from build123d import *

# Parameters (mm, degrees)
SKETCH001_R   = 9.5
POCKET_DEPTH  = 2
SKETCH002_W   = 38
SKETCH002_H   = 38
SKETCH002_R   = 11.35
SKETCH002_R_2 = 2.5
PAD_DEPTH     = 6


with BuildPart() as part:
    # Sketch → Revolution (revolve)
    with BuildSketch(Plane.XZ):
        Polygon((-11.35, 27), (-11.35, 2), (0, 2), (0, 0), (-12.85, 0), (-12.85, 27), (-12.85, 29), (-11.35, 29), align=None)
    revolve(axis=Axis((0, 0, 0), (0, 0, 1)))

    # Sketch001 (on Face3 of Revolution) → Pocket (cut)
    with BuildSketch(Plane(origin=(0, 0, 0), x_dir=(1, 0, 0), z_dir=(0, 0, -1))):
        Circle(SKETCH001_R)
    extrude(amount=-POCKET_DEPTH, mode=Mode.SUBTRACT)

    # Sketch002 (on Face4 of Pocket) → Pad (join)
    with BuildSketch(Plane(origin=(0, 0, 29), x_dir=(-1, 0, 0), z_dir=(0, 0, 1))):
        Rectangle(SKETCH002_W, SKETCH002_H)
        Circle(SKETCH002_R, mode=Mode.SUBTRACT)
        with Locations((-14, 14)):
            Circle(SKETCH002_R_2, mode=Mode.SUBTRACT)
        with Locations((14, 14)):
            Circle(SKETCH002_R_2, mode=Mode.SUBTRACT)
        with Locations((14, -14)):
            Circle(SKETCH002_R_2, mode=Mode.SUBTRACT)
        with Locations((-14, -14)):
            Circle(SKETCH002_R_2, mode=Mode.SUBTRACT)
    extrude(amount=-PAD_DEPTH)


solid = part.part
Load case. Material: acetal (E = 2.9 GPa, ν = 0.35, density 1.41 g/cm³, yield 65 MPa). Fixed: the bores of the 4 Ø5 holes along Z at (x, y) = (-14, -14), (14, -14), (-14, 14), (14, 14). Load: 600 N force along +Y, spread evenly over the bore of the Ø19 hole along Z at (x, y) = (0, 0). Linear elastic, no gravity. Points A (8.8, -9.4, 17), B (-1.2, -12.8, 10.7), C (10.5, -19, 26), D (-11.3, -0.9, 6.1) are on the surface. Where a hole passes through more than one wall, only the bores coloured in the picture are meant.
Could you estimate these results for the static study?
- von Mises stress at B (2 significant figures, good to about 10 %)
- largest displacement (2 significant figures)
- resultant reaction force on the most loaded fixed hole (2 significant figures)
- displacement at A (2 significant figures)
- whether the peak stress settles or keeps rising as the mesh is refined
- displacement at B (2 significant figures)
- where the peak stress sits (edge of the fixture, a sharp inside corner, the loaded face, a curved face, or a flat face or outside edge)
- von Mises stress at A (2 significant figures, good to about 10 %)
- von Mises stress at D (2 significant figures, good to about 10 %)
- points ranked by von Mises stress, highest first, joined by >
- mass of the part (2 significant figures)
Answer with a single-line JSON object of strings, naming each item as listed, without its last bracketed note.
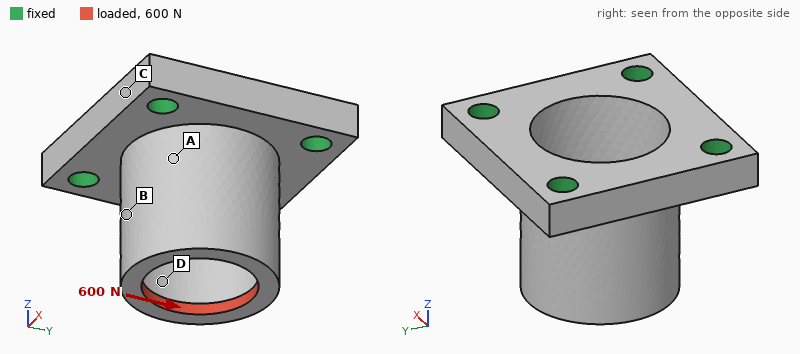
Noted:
{"von Mises stress at B": "8.9 MPa", "largest displacement": "0.58 mm", "resultant reaction force on the most loaded fixed hole": "360 N", "displacement at A": "0.15 mm", "whether the peak stress settles or keeps rising as the mesh is refined": "keeps rising", "displacement at B": "0.31 mm", "where the peak stress sits": "edge of the fixture", "von Mises stress at A": "13 MPa", "von Mises stress at D": "21 MPa", "points ranked by von Mises stress, highest first, joined by >": "D > A > B > C", "mass of the part": "12 g"}
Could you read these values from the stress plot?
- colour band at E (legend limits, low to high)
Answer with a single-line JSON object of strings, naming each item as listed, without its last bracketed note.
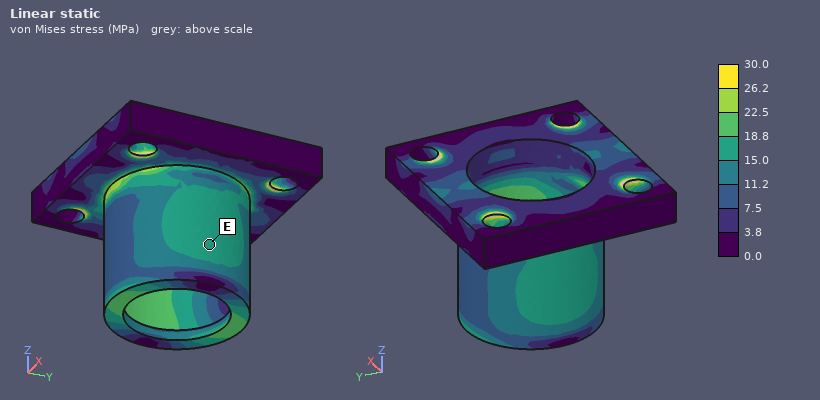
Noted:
{"colour band at E": "15.0 to 18.8 MPa"}
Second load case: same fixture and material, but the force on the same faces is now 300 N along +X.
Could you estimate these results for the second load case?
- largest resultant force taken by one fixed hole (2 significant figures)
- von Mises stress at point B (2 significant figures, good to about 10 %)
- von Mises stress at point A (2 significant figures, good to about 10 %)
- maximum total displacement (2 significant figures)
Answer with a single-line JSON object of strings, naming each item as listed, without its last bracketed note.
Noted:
{"largest resultant force taken by one fixed hole": "180 N", "von Mises stress at point B": "8.9 MPa", "von Mises stress at point A": "6.8 MPa", "maximum total displacement": "0.29 mm"}
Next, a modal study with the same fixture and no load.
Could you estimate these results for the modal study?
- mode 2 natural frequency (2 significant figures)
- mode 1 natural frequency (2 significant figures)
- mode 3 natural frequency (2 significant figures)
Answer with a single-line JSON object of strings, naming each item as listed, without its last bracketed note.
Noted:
{"mode 2 natural frequency": "4000 Hz", "mode 1 natural frequency": "4000 Hz", "mode 3 natural frequency": "4100 Hz"}
